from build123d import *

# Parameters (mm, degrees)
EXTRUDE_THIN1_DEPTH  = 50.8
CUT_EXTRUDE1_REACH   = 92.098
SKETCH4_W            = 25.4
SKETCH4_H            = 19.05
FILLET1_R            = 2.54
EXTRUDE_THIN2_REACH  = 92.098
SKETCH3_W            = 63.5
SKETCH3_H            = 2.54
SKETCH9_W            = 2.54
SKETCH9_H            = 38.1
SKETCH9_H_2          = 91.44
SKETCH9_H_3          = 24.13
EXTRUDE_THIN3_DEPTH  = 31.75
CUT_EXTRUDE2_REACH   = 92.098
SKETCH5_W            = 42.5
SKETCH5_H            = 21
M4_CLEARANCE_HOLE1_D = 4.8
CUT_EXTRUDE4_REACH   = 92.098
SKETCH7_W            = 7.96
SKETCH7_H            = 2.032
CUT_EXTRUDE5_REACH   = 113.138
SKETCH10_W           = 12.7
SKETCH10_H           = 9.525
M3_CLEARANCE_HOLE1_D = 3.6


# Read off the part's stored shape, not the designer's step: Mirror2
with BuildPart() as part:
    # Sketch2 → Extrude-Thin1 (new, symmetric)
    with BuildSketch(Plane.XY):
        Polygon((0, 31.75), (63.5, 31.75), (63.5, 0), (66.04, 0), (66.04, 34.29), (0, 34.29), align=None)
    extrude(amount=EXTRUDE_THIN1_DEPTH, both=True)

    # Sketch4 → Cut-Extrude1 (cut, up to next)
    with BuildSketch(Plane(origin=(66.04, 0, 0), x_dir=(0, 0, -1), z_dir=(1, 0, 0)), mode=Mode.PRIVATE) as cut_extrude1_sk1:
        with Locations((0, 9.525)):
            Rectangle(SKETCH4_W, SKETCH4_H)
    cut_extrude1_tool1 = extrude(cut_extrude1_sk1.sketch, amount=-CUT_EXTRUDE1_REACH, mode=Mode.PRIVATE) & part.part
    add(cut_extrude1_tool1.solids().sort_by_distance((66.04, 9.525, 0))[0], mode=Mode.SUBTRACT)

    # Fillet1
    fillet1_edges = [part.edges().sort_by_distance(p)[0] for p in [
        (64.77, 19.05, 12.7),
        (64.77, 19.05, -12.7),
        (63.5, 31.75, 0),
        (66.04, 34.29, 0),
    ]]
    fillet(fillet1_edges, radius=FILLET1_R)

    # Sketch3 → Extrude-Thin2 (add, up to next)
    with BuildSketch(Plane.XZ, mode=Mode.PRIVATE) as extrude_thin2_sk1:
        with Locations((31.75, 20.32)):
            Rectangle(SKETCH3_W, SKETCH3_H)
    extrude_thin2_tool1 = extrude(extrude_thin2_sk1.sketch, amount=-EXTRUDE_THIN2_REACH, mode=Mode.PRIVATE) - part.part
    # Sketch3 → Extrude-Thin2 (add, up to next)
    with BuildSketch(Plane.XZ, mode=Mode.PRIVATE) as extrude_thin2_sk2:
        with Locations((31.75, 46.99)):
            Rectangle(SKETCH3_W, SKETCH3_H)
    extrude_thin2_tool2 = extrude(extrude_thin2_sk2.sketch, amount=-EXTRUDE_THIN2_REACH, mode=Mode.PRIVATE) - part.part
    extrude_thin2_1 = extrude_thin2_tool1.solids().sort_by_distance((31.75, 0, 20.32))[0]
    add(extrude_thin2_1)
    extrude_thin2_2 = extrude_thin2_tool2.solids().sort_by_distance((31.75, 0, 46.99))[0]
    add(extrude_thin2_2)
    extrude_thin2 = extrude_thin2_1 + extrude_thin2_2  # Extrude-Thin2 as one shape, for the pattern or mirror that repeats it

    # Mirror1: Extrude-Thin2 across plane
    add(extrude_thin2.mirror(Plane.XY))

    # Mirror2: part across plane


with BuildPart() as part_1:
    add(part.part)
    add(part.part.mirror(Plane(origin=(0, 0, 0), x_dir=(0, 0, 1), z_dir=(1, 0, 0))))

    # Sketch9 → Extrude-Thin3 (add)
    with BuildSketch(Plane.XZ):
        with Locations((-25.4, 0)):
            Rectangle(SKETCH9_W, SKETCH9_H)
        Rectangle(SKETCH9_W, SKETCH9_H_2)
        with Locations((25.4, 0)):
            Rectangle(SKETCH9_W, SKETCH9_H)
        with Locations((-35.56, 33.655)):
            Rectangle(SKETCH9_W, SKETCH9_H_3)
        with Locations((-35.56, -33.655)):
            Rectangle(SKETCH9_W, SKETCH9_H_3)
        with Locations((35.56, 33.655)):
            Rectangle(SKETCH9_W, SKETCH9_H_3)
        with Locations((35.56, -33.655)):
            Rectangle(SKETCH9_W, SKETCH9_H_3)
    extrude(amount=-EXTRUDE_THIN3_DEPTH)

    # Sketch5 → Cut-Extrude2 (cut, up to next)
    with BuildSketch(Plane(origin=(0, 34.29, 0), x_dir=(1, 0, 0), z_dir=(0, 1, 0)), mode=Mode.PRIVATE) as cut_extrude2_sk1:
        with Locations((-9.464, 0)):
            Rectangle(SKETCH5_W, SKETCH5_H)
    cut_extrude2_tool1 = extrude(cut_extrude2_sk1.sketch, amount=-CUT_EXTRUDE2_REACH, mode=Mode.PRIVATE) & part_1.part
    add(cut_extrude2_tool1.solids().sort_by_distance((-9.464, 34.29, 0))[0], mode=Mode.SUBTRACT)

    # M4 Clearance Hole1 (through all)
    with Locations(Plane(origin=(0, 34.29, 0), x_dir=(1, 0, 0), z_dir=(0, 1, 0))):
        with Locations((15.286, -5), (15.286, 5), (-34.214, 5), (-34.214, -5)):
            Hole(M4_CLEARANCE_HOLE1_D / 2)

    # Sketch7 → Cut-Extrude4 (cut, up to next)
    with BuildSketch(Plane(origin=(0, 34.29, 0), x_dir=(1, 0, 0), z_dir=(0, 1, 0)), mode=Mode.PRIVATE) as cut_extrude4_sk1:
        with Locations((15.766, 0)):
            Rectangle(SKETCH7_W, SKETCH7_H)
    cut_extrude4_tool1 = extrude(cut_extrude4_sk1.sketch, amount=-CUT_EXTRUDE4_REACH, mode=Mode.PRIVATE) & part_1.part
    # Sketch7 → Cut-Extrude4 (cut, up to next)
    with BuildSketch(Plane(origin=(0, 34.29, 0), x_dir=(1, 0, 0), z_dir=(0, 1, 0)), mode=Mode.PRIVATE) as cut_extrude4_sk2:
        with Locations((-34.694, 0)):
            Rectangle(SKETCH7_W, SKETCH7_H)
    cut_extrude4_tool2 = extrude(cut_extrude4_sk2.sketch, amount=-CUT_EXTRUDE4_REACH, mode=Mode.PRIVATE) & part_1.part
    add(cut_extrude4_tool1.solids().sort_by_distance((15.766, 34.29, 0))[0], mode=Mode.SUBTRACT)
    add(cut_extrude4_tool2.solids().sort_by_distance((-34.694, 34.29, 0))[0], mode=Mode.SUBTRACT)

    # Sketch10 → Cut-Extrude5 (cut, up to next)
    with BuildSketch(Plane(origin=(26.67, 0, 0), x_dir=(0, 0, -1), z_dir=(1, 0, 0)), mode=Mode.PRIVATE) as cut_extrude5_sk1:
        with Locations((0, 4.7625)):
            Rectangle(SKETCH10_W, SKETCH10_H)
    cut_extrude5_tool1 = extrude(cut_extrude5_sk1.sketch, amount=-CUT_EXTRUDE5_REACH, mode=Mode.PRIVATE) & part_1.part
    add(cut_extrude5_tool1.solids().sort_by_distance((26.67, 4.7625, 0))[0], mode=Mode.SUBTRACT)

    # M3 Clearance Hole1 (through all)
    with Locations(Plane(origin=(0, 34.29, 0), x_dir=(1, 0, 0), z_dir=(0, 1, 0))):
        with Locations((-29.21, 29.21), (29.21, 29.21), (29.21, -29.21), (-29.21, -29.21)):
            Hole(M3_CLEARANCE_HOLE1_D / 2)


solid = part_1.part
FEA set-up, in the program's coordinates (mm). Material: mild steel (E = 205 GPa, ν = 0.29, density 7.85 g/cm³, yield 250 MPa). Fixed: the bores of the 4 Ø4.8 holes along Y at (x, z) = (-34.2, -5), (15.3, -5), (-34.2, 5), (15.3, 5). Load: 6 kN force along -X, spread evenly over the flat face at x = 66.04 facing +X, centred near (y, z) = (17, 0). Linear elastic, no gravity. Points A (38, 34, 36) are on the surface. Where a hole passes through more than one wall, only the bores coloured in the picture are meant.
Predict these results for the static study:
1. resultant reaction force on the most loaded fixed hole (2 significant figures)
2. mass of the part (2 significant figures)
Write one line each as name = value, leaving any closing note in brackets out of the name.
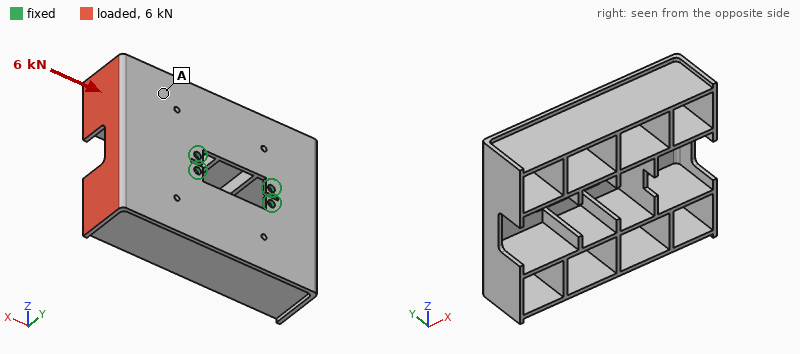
resultant reaction force on the most loaded fixed hole = 2.0 kN
mass of the part = 810 g
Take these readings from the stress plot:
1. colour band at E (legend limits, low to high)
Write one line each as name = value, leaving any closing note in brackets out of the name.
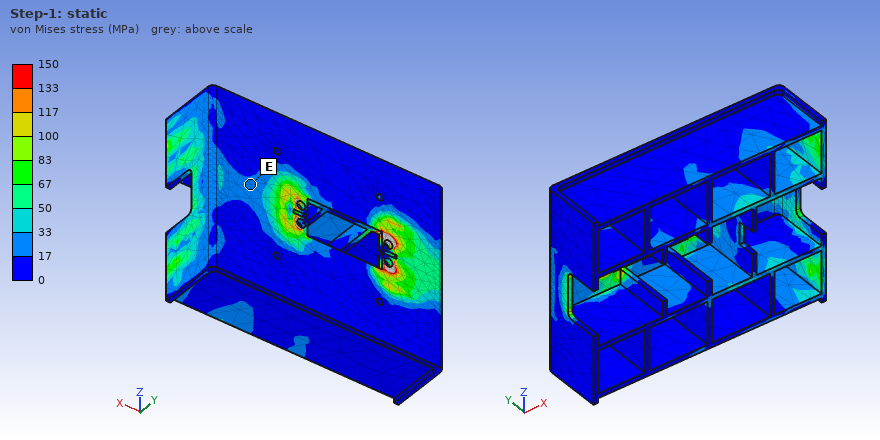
colour band at E = 17 to 33 MPa
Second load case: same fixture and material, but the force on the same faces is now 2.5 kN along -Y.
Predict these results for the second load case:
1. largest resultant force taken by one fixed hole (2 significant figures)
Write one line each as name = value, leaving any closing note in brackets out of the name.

largest resultant force taken by one fixed hole = 2.4 kN
